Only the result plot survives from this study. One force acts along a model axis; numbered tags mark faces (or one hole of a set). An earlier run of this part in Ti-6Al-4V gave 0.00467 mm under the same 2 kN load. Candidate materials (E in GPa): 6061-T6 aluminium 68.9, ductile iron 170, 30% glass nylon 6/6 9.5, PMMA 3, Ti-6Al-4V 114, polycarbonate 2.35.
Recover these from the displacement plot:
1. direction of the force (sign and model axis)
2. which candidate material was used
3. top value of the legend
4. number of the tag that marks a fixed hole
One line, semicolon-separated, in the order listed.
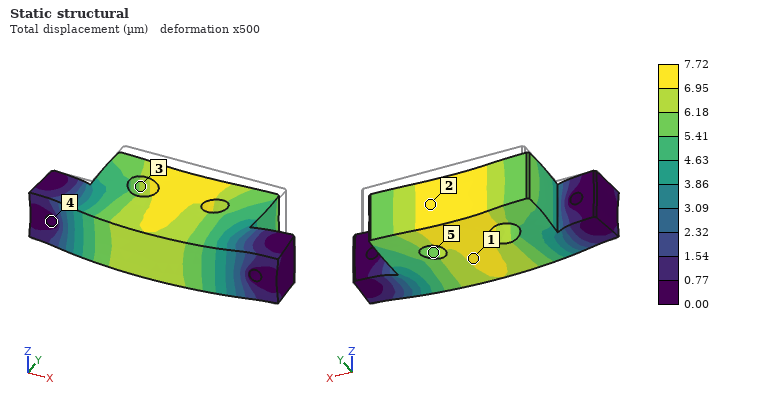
-Y; 6061-T6 aluminium; 7.72 µm; 4
